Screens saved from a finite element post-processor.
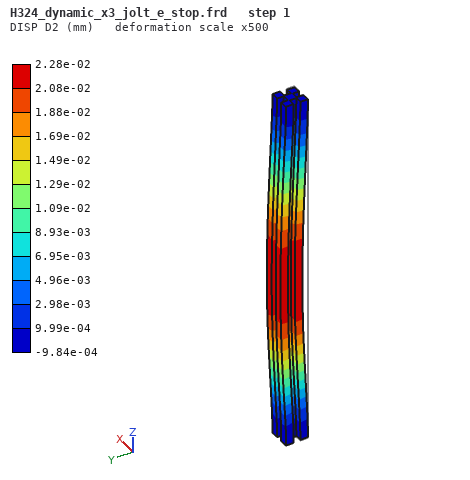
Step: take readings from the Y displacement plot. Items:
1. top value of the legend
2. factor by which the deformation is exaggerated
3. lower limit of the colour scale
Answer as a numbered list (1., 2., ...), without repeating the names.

1. 2.28e-02 mm
2. 500
3. -9.84e-04 mm
